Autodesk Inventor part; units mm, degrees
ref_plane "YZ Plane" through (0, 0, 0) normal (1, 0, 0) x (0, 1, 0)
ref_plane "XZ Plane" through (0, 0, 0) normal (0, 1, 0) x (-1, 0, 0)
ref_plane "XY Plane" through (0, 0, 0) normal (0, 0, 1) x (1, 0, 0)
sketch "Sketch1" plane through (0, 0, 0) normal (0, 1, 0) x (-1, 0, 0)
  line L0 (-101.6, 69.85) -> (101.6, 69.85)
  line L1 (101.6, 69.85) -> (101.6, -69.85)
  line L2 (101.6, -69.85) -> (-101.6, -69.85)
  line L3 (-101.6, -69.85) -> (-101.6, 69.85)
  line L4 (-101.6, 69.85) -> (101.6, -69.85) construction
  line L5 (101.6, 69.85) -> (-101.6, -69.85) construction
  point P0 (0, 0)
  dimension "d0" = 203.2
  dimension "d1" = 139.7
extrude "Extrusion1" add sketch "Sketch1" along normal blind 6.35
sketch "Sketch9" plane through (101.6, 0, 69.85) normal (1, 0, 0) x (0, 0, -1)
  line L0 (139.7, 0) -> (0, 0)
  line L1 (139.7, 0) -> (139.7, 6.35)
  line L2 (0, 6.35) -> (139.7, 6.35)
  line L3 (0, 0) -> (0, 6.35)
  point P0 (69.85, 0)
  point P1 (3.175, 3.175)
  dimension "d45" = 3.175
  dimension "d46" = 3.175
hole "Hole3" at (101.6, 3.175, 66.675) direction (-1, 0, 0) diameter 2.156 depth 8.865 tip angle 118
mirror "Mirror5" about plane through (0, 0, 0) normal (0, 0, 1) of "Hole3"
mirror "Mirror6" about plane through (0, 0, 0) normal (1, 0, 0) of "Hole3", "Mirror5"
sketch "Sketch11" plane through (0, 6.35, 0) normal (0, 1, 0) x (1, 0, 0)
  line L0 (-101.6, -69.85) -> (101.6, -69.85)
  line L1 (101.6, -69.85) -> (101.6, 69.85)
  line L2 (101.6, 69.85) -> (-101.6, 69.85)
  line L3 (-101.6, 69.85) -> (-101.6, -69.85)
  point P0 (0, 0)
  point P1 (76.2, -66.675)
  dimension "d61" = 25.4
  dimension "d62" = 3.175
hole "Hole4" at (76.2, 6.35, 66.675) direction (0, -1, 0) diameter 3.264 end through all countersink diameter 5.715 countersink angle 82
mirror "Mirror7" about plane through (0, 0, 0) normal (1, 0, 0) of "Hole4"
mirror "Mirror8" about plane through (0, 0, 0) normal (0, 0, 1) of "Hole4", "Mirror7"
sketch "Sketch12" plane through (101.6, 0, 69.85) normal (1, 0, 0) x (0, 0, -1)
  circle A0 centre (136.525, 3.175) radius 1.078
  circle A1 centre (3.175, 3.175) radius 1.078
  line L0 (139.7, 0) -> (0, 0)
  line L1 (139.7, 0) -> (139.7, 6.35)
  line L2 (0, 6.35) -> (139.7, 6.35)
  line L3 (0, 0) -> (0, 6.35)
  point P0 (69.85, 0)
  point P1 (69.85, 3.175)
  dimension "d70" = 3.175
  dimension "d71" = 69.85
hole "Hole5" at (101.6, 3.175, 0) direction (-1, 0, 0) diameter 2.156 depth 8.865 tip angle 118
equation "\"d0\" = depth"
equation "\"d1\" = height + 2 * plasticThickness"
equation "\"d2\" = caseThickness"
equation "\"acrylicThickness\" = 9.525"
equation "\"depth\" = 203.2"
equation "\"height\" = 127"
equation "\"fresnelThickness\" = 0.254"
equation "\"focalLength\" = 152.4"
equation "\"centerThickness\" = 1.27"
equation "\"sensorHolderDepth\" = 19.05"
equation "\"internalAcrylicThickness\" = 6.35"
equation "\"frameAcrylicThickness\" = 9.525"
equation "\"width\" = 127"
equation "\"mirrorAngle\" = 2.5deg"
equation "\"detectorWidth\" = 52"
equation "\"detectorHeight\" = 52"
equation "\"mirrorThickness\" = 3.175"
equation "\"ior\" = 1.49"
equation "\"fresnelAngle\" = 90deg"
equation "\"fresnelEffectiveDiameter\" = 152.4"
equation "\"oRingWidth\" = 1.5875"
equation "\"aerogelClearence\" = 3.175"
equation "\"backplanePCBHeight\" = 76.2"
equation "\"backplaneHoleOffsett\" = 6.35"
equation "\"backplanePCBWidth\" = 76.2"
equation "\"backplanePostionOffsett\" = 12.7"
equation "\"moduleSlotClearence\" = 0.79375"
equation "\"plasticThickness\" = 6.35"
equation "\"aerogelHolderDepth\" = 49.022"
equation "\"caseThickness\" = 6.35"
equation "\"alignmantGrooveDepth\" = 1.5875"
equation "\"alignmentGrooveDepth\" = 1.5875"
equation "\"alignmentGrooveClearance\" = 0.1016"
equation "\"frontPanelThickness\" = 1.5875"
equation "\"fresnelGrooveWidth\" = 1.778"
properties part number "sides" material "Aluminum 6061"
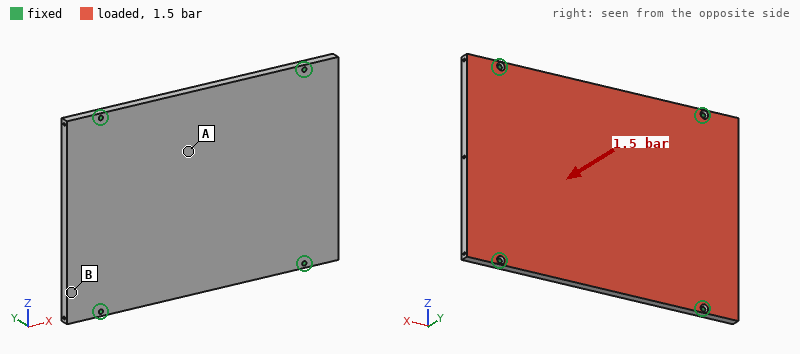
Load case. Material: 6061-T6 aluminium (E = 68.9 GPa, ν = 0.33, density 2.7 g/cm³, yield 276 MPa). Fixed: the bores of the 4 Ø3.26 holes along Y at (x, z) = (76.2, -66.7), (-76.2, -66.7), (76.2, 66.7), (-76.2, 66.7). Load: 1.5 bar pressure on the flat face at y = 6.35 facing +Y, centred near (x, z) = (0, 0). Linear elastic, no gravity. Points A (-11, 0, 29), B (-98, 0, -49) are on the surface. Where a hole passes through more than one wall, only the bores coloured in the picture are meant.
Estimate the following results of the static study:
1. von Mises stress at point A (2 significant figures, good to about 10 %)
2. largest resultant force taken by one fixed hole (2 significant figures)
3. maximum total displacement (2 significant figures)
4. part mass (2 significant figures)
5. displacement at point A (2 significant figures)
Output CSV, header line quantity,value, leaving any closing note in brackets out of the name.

quantity,value
von Mises stress at point A,29 MPa
largest resultant force taken by one fixed hole,1.1 kN
maximum total displacement,0.43 mm
part mass,490 g
displacement at point A,0.39 mm
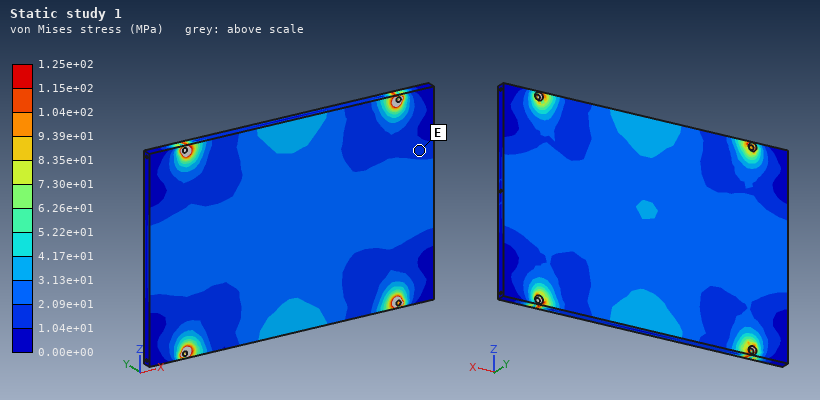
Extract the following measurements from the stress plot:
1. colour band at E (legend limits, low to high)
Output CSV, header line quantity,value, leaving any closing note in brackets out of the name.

quantity,value
colour band at E,1.04e+01 to 2.09e+01 MPa
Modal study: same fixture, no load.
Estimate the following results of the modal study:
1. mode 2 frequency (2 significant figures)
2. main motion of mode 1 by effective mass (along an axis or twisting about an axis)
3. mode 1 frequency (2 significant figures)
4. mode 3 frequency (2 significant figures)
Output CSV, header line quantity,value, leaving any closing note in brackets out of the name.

quantity,value
mode 2 frequency,1500 Hz
main motion of mode 1 by effective mass,along Y
mode 1 frequency,840 Hz
mode 3 frequency,1500 Hz
